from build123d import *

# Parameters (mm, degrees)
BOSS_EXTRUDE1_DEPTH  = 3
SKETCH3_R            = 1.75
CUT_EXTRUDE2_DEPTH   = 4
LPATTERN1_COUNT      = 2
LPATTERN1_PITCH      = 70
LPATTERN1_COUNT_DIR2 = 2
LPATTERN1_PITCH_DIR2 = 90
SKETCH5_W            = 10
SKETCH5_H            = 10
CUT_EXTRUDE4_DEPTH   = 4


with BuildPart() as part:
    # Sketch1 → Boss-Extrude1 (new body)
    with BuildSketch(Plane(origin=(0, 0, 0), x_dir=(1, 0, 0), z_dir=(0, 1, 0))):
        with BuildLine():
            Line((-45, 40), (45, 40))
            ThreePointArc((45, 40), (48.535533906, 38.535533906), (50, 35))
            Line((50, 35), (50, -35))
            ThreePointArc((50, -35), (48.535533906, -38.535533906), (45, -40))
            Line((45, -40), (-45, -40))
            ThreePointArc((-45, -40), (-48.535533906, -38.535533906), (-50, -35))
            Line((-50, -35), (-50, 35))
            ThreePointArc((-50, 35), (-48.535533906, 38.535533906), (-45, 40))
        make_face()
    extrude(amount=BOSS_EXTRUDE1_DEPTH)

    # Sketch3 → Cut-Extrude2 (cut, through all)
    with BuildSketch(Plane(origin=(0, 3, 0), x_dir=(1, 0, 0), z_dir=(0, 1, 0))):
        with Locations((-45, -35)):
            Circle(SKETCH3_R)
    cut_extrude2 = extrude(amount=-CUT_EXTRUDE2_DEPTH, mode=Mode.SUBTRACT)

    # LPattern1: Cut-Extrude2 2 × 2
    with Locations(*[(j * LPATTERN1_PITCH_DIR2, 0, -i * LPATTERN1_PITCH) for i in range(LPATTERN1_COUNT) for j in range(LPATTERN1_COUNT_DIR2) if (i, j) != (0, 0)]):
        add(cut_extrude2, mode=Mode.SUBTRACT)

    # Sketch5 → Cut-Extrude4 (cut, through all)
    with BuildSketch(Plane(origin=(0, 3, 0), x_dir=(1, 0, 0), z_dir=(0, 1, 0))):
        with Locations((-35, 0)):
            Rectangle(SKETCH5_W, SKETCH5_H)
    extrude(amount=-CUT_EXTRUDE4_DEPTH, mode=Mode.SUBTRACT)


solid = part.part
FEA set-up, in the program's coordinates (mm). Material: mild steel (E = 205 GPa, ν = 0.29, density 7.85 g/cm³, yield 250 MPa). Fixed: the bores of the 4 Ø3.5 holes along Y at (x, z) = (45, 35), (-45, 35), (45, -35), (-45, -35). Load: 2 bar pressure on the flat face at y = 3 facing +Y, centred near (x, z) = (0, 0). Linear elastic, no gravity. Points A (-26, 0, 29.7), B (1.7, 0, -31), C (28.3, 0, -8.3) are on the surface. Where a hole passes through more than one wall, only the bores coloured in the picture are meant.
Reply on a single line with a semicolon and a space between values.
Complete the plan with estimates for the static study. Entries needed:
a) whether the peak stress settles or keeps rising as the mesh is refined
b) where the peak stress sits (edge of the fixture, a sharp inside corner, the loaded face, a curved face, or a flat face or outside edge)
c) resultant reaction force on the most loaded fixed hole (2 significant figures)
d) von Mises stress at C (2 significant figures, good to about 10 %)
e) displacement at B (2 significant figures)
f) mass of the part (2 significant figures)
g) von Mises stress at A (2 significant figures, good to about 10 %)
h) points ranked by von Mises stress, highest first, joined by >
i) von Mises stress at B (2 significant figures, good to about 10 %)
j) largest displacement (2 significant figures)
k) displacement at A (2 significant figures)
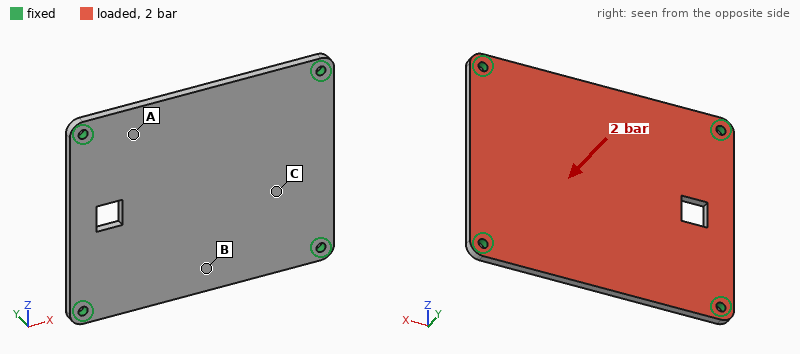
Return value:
keeps rising; edge of the fixture; 400 N; 34 MPa; 0.12 mm; 180 g; 18 MPa; B > C > A; 59 MPa; 0.15 mm; 0.064 mm
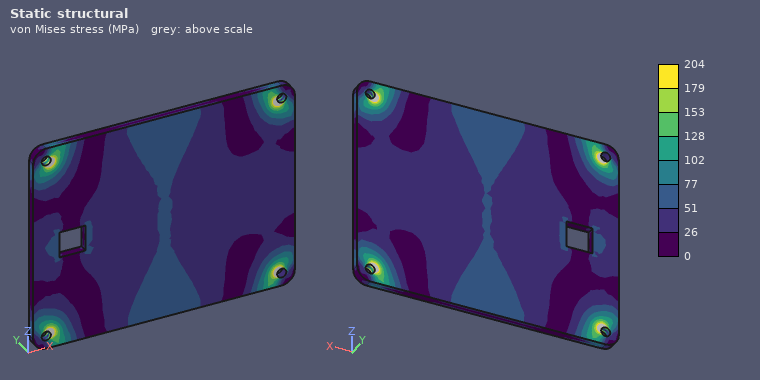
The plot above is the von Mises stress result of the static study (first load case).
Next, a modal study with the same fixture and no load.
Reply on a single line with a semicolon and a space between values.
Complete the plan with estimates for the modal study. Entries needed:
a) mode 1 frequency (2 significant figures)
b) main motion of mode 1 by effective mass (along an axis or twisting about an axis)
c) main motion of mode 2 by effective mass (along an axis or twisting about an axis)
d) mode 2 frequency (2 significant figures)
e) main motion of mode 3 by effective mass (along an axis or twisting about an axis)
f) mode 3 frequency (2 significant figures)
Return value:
1400 Hz; along Y; twisting about X; 2300 Hz; twisting about Z; 3100 Hz
